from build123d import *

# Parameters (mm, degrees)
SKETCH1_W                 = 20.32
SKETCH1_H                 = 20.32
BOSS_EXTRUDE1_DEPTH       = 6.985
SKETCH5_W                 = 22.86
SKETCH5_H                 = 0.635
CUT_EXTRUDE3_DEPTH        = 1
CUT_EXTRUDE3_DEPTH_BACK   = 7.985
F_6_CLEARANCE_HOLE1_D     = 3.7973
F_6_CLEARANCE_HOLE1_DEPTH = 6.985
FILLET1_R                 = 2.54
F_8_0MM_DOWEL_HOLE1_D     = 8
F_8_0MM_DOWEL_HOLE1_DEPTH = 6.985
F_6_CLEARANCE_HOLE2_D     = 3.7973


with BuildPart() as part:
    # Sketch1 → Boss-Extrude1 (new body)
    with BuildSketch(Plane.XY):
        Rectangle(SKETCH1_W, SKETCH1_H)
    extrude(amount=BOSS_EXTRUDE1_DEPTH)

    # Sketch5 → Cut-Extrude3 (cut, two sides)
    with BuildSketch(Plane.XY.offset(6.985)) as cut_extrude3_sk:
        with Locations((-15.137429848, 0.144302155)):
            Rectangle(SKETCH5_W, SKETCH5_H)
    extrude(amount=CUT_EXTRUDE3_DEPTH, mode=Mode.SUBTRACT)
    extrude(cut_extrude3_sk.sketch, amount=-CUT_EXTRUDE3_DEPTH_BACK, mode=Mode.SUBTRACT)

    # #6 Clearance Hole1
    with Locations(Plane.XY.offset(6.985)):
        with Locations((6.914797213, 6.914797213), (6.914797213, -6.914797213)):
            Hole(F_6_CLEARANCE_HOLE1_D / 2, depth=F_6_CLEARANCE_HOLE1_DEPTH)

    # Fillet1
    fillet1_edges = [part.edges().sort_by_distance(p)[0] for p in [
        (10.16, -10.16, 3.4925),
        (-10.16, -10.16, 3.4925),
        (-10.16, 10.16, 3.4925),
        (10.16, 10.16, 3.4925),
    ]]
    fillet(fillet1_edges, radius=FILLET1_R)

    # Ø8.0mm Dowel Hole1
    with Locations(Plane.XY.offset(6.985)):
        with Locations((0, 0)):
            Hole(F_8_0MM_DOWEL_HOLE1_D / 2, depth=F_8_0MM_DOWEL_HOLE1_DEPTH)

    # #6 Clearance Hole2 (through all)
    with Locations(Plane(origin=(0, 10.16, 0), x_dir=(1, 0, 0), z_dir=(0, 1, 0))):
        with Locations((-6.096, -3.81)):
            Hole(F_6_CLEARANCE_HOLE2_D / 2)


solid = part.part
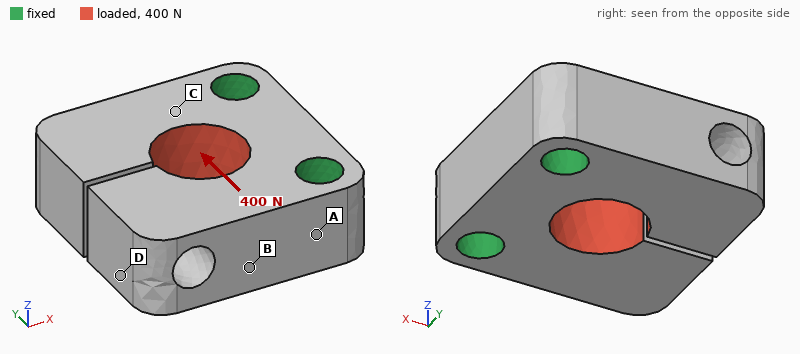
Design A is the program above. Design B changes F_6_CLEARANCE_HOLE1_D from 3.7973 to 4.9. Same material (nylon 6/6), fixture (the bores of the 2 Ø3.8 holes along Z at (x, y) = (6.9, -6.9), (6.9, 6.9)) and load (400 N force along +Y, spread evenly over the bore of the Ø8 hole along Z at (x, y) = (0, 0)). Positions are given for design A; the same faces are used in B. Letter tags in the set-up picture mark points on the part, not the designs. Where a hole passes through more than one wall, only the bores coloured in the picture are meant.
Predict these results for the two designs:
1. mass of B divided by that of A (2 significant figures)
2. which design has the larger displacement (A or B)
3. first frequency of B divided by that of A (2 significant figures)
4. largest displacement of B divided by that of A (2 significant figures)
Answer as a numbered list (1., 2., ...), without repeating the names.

1. 0.95
2. A
3. 1.1
4. 0.88
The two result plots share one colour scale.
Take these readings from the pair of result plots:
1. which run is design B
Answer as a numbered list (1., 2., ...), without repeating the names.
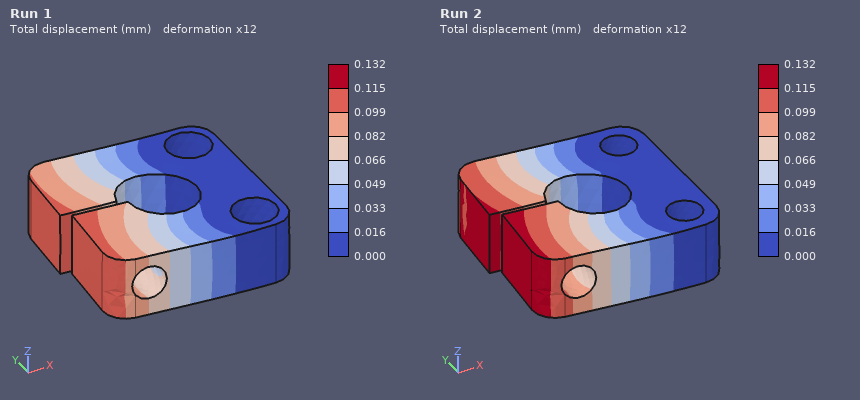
1. Run 1
